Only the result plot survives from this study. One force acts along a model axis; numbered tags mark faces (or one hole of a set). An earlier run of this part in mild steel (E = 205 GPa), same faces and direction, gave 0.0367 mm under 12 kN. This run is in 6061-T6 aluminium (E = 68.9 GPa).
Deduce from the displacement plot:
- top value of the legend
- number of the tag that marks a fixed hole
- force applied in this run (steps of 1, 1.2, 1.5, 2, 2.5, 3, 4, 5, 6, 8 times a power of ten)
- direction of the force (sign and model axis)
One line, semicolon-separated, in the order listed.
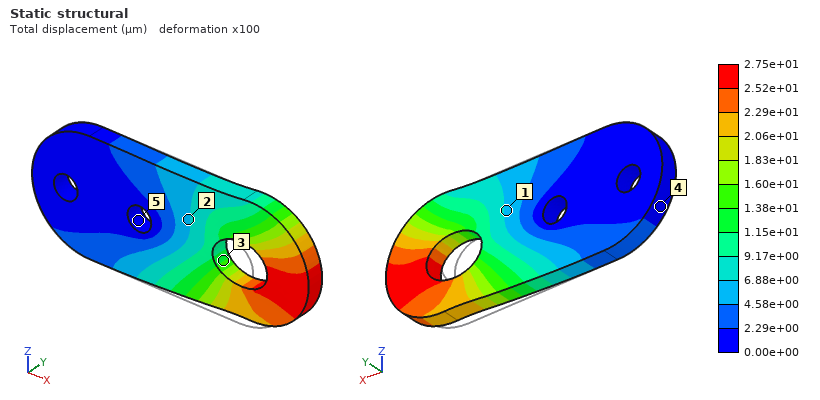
2.75e+01 µm; 5; 3 kN; +X
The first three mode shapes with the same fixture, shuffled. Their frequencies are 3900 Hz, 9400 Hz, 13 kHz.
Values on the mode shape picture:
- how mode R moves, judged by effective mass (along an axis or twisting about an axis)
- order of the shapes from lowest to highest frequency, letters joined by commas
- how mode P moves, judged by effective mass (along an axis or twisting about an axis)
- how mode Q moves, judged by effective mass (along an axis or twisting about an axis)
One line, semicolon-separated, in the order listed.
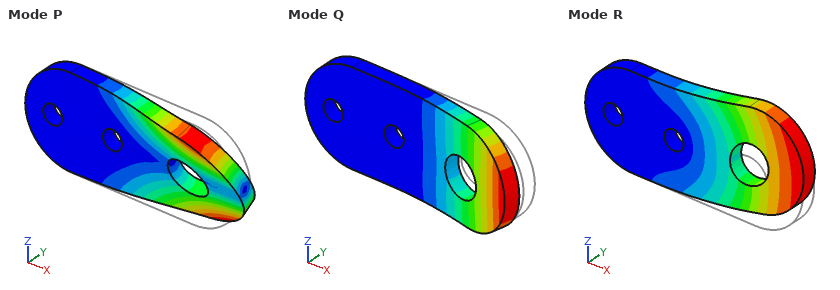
along Z; Q, P, R; twisting about X; along Y
